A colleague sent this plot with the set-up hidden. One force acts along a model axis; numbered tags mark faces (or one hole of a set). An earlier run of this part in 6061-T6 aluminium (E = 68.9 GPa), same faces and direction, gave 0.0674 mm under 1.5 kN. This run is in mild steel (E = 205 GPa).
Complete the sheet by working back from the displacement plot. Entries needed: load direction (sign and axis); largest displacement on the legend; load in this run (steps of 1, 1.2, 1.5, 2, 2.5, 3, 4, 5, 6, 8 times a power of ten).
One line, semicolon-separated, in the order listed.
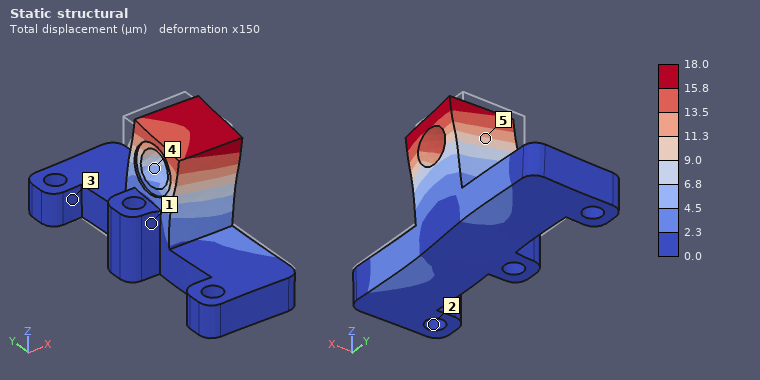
-Y; 18.0 µm; 1.2 kN
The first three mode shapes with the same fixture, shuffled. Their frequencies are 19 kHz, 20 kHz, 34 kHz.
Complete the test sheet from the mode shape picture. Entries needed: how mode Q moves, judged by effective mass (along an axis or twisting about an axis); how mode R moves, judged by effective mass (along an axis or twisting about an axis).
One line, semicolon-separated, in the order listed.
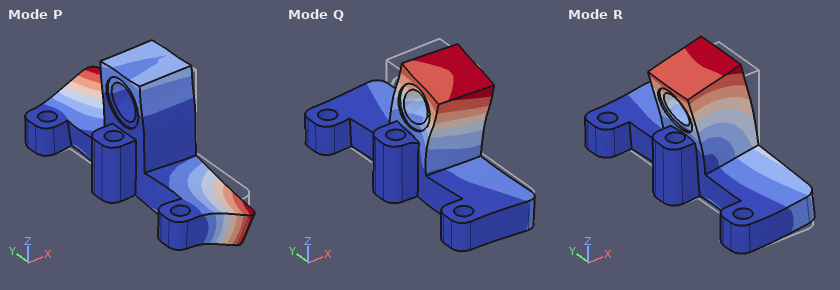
along Y; along Z
